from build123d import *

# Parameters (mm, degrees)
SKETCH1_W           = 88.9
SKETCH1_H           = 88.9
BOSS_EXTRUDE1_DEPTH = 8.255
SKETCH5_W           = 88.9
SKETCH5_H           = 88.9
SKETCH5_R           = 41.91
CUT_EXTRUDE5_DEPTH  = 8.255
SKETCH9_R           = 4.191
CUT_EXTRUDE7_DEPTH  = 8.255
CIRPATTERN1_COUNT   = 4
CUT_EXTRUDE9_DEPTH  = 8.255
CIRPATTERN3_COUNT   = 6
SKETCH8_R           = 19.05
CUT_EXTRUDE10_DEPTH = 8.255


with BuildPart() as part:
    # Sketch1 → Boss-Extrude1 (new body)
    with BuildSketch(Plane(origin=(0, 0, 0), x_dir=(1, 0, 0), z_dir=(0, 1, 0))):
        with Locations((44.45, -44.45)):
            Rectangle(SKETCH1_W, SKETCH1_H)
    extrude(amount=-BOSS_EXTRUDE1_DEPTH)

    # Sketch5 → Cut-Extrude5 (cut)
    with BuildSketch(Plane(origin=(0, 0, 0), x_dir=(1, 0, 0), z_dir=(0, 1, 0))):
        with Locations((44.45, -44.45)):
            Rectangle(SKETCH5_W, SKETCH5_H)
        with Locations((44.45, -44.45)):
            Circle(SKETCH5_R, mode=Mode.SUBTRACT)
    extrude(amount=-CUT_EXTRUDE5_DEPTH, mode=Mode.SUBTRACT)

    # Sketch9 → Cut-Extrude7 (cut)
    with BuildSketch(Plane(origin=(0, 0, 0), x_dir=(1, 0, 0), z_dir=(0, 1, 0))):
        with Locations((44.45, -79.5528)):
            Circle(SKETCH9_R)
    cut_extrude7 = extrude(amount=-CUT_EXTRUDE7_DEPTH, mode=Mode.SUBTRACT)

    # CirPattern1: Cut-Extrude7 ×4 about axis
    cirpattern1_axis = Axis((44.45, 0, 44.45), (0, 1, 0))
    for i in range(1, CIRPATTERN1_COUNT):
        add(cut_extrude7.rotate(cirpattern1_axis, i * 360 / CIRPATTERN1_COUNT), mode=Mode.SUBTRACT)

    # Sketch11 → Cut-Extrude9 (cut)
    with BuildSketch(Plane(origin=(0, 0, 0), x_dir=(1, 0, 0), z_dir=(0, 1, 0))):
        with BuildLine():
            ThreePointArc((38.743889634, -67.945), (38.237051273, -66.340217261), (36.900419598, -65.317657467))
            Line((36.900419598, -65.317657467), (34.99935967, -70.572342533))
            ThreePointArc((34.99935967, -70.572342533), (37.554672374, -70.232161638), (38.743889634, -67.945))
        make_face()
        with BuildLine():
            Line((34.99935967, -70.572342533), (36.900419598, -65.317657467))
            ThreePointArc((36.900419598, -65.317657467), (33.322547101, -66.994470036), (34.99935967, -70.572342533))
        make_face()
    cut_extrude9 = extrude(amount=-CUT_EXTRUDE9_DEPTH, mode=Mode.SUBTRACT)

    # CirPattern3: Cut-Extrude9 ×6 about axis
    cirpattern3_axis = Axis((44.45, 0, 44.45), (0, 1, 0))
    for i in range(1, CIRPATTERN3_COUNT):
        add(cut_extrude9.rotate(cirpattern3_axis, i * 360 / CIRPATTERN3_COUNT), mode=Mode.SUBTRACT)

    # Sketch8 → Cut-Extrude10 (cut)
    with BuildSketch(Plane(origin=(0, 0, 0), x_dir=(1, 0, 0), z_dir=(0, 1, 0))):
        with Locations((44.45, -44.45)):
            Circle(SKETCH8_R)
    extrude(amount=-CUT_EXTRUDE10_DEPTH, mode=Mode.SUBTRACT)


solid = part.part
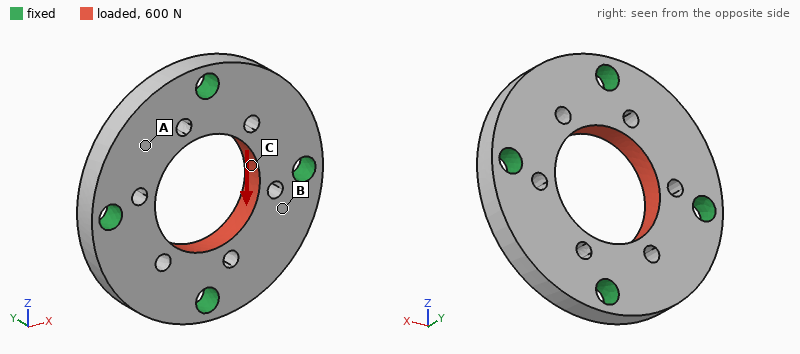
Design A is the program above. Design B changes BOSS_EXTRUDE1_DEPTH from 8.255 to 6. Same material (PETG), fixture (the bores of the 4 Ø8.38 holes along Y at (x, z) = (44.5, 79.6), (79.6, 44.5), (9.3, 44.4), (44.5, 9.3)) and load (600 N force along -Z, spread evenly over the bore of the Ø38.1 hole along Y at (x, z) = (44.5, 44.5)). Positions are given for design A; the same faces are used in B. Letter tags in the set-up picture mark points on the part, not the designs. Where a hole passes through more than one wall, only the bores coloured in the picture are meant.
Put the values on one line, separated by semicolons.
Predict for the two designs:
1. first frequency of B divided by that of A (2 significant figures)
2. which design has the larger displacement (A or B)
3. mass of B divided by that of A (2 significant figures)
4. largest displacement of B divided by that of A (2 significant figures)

0.80; B; 0.73; 1.4
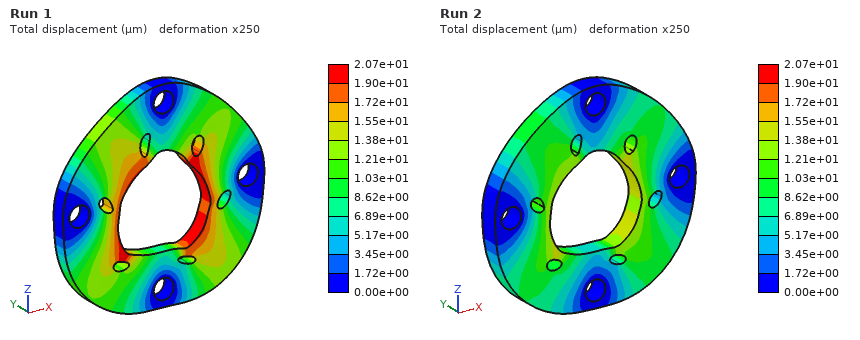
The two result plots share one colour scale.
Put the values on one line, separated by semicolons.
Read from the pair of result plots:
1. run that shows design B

Run 1
